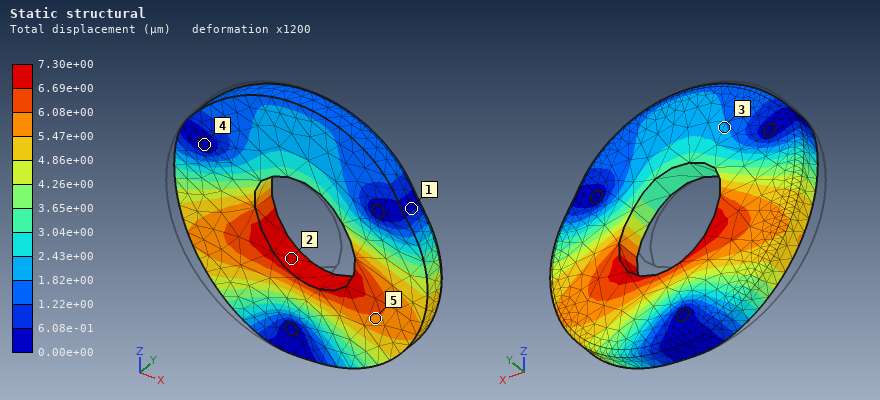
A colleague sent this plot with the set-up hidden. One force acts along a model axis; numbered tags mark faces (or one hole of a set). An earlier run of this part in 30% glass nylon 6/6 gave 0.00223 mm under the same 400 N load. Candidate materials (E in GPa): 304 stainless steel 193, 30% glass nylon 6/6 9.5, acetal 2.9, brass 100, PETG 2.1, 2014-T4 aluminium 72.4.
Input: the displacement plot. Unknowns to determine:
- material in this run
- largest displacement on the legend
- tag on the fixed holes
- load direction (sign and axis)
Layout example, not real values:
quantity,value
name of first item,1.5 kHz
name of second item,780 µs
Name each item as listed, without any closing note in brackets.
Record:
quantity,value
material in this run,acetal
largest displacement on the legend,7.30e+00 µm
tag on the fixed holes,4
load direction,+X
